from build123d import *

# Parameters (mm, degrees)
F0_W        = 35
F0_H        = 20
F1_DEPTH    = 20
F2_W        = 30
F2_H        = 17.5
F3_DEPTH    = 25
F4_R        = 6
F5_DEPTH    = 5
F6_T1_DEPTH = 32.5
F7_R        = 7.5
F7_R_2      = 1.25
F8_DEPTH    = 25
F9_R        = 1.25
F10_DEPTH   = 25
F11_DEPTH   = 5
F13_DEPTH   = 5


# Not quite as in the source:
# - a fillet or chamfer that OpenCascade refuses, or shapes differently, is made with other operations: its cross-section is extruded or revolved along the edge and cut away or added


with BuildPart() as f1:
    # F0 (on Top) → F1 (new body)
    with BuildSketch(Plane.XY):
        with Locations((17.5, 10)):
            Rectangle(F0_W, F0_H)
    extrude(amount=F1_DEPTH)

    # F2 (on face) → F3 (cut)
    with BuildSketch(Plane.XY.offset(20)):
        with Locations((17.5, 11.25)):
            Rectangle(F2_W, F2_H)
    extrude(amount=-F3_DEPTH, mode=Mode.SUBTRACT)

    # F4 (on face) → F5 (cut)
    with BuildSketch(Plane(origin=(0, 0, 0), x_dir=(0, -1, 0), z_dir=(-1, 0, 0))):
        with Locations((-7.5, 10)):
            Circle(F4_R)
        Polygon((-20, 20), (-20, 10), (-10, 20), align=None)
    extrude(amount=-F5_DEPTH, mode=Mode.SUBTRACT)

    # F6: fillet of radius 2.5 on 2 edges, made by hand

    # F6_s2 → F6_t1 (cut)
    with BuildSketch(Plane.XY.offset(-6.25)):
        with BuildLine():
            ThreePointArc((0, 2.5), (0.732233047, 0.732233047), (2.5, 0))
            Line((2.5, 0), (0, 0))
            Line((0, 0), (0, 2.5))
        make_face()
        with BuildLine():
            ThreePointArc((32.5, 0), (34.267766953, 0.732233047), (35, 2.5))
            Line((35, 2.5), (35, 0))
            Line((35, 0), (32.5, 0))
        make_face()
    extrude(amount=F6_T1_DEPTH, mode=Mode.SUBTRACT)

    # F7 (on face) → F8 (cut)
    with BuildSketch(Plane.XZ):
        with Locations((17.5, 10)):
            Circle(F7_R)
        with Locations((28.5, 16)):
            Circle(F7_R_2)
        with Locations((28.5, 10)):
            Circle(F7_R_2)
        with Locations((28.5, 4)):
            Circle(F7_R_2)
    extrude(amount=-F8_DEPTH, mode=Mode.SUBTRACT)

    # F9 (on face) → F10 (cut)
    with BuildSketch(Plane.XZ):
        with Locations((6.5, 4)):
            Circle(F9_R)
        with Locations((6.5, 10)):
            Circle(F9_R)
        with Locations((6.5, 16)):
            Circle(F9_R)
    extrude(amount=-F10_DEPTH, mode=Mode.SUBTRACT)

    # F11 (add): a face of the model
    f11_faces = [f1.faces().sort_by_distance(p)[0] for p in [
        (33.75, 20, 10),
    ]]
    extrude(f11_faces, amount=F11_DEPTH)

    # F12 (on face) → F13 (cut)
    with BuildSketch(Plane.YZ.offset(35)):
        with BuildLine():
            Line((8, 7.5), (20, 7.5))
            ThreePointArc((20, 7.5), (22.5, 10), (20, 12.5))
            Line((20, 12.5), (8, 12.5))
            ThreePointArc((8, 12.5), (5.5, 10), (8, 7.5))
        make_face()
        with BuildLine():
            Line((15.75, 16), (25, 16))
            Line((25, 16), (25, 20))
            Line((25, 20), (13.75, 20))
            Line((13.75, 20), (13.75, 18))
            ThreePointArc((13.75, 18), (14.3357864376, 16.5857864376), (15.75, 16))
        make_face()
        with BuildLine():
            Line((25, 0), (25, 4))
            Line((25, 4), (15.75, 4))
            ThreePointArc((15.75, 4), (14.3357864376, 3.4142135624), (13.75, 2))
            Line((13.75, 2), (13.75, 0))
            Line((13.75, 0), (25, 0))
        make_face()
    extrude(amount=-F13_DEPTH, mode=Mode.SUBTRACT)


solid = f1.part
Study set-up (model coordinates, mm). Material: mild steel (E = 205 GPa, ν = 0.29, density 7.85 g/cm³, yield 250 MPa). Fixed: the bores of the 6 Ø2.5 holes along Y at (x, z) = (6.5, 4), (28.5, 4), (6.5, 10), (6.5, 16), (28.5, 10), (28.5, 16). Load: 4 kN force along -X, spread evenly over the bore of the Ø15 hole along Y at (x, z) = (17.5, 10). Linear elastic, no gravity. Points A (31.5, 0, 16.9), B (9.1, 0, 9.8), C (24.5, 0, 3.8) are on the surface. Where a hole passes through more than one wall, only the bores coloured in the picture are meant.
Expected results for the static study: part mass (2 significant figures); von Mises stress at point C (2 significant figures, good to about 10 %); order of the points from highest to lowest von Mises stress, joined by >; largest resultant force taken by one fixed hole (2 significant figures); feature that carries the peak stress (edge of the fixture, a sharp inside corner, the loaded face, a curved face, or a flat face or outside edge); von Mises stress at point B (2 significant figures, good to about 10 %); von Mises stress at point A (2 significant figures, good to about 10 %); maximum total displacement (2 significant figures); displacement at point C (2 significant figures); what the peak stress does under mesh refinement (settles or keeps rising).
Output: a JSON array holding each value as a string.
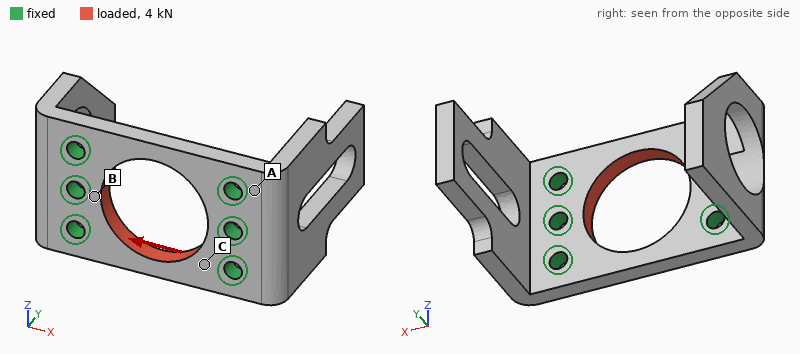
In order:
["18 g", "60 MPa", "C > B > A", "790 N", "edge of the fixture", "36 MPa", "12 MPa", "2.6 µm", "0.98 µm", "keeps rising"]
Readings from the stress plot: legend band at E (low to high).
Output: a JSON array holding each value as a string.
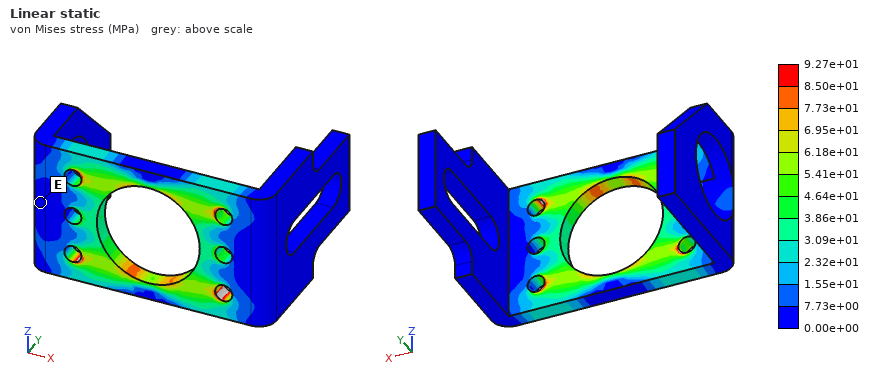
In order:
["0.00e+00 to 7.73e+00 MPa"]
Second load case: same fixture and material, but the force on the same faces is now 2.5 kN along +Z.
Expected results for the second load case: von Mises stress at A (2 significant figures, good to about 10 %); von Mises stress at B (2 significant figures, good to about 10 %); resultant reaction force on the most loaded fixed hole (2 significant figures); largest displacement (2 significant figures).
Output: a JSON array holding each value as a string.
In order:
["10 MPa", "49 MPa", "550 N", "6.7 µm"]
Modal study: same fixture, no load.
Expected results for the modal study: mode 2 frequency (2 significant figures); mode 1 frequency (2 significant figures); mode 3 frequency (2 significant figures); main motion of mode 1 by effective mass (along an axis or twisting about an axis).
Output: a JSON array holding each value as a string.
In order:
["4000 Hz", "3800 Hz", "9700 Hz", "along X"]
